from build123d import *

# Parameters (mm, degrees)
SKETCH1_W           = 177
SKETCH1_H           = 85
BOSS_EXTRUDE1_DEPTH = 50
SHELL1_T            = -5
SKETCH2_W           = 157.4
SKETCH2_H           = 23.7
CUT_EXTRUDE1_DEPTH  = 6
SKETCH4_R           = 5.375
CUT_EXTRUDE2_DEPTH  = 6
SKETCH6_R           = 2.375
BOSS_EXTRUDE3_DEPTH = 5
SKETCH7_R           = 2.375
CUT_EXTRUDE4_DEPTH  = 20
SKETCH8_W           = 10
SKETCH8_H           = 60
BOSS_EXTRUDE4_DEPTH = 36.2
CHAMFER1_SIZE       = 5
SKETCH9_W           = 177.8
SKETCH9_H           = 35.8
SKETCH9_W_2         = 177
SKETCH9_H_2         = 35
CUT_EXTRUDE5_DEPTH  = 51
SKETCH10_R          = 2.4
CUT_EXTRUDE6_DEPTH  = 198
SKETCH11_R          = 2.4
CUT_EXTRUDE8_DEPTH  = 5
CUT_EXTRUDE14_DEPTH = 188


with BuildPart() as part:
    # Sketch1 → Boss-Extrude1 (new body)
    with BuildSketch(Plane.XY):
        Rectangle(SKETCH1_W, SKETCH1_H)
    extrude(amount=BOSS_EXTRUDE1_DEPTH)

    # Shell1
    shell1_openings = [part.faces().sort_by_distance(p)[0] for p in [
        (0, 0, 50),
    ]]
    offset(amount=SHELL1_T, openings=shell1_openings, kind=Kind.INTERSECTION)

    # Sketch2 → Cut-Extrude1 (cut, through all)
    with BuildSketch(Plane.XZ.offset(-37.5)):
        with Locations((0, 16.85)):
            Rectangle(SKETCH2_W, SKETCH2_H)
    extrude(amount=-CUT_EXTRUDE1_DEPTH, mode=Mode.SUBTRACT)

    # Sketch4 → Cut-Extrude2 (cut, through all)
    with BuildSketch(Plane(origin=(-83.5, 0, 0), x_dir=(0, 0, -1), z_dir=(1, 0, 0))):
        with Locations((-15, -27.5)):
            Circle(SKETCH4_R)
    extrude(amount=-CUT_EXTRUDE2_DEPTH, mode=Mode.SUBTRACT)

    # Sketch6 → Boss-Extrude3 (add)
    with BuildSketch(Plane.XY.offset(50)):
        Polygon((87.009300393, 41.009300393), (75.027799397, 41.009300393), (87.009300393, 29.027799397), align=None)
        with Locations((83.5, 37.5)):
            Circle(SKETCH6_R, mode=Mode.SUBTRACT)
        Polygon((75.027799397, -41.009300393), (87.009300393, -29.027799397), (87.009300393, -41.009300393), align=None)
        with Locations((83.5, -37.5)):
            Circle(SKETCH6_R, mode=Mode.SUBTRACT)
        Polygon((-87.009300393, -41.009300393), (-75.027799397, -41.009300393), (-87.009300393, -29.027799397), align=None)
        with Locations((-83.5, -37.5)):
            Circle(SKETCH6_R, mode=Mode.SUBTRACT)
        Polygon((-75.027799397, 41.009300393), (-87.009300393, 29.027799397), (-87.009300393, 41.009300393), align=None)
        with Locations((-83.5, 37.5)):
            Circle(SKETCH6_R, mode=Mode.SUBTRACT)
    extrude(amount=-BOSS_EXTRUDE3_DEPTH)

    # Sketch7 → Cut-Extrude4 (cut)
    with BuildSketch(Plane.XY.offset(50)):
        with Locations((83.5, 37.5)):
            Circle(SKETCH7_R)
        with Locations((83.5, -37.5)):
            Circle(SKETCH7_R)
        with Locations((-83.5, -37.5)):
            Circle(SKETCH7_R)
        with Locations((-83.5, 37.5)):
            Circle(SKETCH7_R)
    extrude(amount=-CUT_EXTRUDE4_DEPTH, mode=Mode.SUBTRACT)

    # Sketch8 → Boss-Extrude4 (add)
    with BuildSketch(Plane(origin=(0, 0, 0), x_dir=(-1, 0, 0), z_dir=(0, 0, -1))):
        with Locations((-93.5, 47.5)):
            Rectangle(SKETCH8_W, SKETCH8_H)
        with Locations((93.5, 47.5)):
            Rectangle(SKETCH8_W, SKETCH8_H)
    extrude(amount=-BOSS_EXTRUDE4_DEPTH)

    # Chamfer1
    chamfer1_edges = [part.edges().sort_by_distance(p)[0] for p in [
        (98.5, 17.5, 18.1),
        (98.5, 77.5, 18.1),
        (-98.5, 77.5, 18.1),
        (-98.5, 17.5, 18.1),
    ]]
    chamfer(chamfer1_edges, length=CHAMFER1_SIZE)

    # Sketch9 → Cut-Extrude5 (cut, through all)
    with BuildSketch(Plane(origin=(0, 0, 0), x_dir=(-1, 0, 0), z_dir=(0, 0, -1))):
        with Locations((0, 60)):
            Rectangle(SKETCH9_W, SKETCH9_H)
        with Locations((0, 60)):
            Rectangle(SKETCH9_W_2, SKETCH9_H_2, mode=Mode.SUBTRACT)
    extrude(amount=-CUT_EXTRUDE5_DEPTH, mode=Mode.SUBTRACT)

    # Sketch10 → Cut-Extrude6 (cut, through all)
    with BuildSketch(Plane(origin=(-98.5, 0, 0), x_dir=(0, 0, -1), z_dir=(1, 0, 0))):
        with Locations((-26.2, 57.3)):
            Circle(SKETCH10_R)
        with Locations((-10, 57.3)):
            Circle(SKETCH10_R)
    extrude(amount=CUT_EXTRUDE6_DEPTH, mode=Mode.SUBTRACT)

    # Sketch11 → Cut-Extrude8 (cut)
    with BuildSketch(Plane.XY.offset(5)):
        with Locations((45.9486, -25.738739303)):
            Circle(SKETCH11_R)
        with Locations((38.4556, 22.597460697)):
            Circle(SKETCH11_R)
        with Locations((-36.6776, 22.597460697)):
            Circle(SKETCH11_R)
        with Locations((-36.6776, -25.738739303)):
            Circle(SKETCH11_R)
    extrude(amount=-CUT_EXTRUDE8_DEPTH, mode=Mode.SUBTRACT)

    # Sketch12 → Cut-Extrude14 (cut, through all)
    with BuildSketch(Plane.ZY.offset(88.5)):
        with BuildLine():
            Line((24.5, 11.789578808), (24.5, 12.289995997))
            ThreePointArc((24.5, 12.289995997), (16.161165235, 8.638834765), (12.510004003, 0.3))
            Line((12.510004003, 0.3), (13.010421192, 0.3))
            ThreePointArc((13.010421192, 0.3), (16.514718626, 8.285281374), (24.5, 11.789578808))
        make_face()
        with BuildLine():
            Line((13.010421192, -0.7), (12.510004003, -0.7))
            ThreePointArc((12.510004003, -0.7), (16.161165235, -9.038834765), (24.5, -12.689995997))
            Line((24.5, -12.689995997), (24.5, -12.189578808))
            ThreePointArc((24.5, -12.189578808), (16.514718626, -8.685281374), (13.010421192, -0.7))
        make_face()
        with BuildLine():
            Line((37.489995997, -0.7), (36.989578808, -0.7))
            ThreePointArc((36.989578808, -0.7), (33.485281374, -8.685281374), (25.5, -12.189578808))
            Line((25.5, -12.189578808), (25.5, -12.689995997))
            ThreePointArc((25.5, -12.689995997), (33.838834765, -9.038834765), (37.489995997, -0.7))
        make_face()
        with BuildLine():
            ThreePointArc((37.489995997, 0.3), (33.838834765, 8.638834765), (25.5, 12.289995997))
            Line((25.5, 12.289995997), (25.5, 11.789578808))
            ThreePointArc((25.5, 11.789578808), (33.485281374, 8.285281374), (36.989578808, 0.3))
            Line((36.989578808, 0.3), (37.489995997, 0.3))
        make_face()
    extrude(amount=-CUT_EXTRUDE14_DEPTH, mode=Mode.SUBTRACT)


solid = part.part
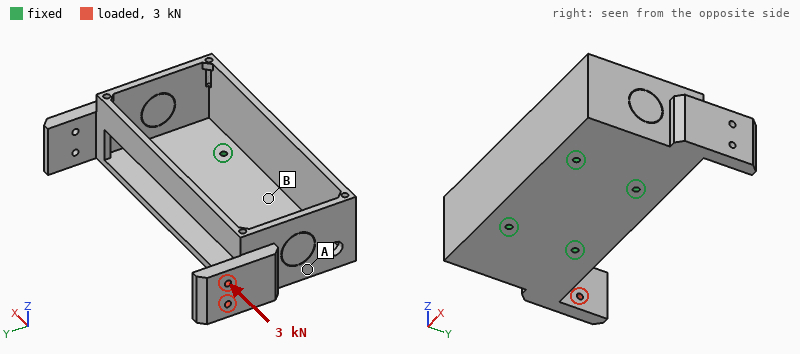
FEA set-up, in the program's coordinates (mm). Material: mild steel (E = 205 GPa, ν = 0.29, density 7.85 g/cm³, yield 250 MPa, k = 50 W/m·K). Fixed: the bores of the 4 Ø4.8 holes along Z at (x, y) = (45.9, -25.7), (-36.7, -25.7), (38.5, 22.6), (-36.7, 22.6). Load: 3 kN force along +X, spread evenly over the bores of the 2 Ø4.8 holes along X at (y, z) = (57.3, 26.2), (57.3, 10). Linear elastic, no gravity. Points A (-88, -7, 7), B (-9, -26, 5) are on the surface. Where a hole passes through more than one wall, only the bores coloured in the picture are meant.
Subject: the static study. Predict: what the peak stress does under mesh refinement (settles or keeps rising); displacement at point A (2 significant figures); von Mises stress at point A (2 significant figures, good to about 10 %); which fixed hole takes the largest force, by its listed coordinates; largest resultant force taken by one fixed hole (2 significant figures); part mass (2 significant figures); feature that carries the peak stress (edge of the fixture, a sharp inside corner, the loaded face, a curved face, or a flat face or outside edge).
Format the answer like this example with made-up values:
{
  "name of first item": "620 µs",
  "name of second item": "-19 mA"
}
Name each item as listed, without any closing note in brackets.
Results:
{
  "what the peak stress does under mesh refinement": "keeps rising",
  "displacement at point A": "0.032 mm",
  "von Mises stress at point A": "23 MPa",
  "which fixed hole takes the largest force, by its listed coordinates": "(-36.7, 22.6)",
  "largest resultant force taken by one fixed hole": "3.1 kN",
  "part mass": "1.6 kg",
  "feature that carries the peak stress": "a sharp inside corner"
}
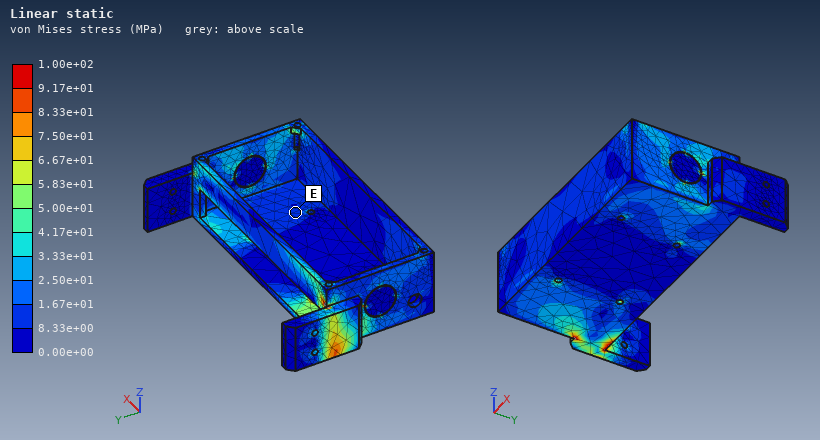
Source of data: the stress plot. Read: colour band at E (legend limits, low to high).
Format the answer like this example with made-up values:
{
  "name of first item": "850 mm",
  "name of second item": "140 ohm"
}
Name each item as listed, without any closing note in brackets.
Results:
{
  "colour band at E": "8.33e+00 to 1.67e+01 MPa"
}
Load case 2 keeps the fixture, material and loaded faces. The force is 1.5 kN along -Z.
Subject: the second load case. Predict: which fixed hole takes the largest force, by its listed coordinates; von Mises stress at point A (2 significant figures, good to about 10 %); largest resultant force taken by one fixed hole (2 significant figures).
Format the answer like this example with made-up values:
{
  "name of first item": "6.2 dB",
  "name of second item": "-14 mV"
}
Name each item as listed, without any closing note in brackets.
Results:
{
  "which fixed hole takes the largest force, by its listed coordinates": "(-36.7, 22.6)",
  "von Mises stress at point A": "59 MPa",
  "largest resultant force taken by one fixed hole": "2.3 kN"
}
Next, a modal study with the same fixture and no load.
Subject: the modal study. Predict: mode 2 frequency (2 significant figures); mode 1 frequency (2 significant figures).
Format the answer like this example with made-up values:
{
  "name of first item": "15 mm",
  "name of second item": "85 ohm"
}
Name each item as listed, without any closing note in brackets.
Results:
{
  "mode 2 frequency": "640 Hz",
  "mode 1 frequency": "560 Hz"
}
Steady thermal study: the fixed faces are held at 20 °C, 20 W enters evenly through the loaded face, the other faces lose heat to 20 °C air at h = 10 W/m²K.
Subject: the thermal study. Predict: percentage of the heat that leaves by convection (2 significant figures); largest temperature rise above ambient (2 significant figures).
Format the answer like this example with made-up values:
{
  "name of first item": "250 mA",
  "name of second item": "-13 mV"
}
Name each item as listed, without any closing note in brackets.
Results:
{
  "percentage of the heat that leaves by convection": "47 %",
  "largest temperature rise above ambient": "70 K"
}
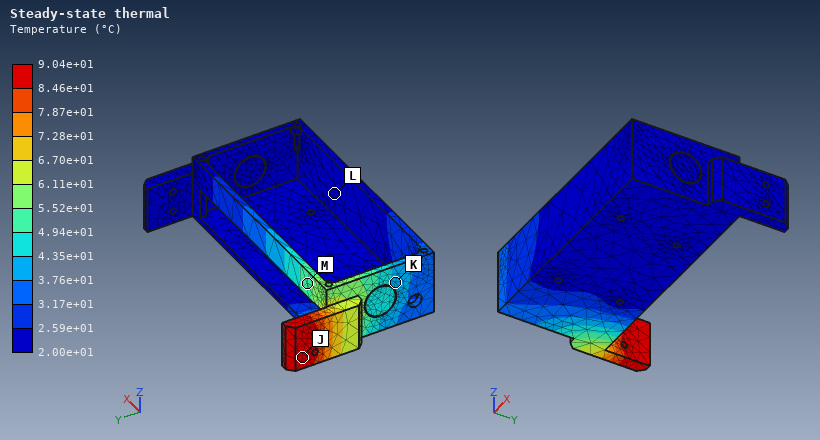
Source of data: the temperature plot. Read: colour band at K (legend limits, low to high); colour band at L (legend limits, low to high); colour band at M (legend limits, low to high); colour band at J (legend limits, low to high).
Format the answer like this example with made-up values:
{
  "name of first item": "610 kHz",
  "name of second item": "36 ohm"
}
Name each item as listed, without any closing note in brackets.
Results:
{
  "colour band at K": "3.76e+01 to 4.35e+01 °C",
  "colour band at L": "2.00e+01 to 2.59e+01 °C",
  "colour band at M": "4.94e+01 to 5.52e+01 °C",
  "colour band at J": "8.46e+01 to 9.04e+01 °C"
}
